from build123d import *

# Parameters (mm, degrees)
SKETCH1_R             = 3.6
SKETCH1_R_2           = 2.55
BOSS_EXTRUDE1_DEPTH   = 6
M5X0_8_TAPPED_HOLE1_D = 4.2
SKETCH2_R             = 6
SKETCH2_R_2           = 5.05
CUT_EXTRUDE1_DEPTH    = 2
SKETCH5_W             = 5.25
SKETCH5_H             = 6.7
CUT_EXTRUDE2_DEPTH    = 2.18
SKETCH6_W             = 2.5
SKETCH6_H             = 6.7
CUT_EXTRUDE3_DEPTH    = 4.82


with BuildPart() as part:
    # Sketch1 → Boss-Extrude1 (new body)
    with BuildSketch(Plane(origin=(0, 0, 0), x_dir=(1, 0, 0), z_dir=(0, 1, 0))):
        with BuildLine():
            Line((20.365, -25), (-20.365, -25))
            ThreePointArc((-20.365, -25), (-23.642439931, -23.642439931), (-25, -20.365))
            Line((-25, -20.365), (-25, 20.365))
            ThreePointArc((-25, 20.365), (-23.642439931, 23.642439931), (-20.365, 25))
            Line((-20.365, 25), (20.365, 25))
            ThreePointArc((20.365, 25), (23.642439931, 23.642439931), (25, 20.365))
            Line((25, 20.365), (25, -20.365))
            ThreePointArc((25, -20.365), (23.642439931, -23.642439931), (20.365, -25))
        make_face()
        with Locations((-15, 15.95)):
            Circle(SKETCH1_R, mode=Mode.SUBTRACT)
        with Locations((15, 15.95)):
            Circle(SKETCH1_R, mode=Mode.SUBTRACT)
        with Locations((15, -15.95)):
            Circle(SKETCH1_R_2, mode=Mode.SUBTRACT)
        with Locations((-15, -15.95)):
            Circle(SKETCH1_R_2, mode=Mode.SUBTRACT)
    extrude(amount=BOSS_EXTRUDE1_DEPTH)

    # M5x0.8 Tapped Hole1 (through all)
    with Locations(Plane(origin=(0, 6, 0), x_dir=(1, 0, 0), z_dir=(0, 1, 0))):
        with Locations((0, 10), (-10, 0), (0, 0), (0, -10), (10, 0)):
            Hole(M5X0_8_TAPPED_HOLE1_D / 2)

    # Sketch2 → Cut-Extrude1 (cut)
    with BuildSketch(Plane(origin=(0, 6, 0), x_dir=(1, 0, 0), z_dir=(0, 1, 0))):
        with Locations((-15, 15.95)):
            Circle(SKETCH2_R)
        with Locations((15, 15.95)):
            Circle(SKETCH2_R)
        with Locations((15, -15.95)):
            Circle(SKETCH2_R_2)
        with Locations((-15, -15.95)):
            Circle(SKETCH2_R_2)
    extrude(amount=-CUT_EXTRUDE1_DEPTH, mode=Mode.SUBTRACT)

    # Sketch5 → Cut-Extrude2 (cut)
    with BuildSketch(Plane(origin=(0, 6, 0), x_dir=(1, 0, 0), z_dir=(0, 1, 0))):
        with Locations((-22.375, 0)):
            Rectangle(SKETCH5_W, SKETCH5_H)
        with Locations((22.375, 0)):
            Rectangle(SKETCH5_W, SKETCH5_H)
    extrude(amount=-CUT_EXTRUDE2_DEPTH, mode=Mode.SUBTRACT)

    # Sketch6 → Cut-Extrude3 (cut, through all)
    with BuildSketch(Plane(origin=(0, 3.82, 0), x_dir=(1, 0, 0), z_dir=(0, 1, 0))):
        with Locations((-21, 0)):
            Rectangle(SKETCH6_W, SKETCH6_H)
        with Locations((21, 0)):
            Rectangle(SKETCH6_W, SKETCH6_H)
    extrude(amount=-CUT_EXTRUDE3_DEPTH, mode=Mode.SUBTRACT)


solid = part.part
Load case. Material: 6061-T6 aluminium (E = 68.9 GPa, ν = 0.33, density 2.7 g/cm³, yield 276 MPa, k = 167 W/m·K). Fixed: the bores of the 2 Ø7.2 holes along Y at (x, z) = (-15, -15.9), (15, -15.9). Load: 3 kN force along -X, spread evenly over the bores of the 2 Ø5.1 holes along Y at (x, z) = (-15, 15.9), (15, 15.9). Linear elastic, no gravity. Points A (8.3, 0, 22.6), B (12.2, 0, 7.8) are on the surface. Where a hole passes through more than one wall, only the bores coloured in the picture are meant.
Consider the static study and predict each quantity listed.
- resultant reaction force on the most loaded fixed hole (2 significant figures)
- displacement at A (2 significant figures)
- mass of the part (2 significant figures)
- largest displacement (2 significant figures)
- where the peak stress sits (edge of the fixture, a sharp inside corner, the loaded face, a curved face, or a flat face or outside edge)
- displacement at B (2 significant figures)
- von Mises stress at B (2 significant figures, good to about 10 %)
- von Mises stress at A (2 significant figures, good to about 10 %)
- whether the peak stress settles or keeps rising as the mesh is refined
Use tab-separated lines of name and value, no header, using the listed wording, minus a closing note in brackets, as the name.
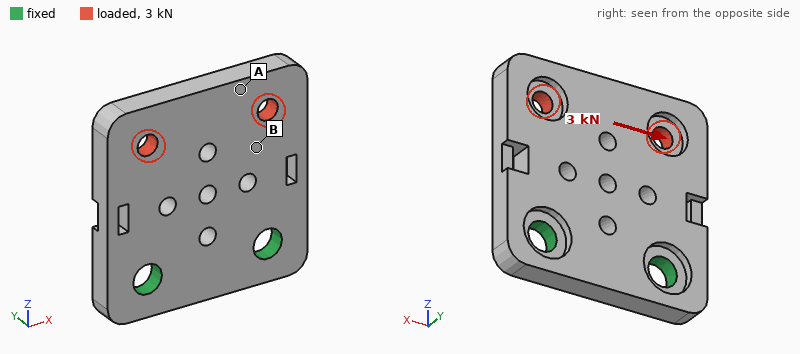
resultant reaction force on the most loaded fixed hole	3.1 kN
displacement at A	41 µm
mass of the part	35 g
largest displacement	54 µm
where the peak stress sits	edge of the fixture
displacement at B	27 µm
von Mises stress at B	40 MPa
von Mises stress at A	10 MPa
whether the peak stress settles or keeps rising as the mesh is refined	keeps rising
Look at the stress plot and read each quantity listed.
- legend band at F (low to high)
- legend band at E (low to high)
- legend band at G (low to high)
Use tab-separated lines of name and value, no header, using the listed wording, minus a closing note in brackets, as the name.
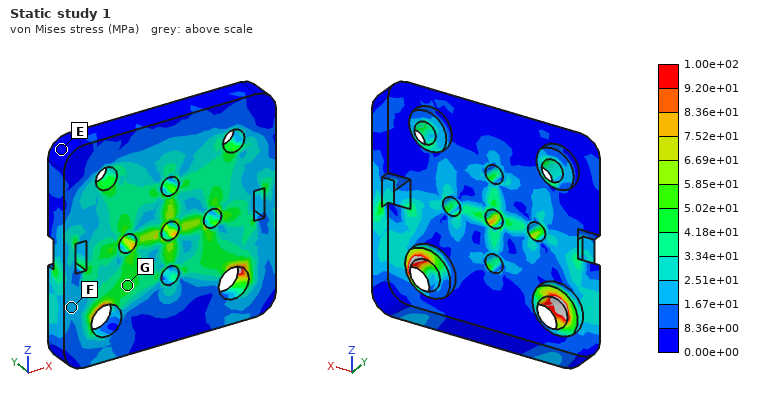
legend band at F	1.67e+01 to 2.51e+01 MPa
legend band at E	0.00e+00 to 8.36e+00 MPa
legend band at G	4.18e+01 to 5.02e+01 MPa
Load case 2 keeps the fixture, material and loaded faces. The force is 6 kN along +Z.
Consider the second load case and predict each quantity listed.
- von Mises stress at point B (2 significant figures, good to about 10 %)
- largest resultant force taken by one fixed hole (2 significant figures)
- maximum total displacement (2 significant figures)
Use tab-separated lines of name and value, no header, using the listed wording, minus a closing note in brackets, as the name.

von Mises stress at point B	45 MPa
largest resultant force taken by one fixed hole	3.0 kN
maximum total displacement	69 µm
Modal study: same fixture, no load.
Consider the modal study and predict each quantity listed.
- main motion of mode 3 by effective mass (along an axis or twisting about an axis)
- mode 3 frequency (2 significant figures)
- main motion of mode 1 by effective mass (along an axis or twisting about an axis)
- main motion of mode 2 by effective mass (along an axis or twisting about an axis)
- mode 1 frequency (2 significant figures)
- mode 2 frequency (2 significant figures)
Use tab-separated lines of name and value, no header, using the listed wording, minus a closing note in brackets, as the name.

main motion of mode 3 by effective mass	along X
mode 3 frequency	12 kHz
main motion of mode 1 by effective mass	along Y
main motion of mode 2 by effective mass	twisting about Z
mode 1 frequency	2600 Hz
mode 2 frequency	5400 Hz
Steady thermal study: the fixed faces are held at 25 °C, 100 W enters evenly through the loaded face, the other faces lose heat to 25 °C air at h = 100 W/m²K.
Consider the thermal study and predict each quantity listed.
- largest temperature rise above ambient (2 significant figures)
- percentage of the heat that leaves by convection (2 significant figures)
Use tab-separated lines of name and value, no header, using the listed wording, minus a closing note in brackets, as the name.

largest temperature rise above ambient	78 K
percentage of the heat that leaves by convection	22 %
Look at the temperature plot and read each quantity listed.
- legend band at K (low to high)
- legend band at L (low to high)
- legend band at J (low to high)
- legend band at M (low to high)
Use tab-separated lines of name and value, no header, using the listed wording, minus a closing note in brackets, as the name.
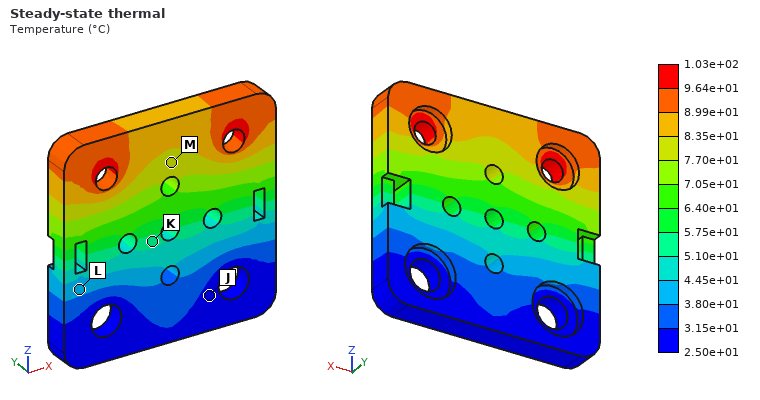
legend band at K	5.10e+01 to 5.75e+01 °C
legend band at L	3.80e+01 to 4.45e+01 °C
legend band at J	2.50e+01 to 3.15e+01 °C
legend band at M	7.70e+01 to 8.35e+01 °C
